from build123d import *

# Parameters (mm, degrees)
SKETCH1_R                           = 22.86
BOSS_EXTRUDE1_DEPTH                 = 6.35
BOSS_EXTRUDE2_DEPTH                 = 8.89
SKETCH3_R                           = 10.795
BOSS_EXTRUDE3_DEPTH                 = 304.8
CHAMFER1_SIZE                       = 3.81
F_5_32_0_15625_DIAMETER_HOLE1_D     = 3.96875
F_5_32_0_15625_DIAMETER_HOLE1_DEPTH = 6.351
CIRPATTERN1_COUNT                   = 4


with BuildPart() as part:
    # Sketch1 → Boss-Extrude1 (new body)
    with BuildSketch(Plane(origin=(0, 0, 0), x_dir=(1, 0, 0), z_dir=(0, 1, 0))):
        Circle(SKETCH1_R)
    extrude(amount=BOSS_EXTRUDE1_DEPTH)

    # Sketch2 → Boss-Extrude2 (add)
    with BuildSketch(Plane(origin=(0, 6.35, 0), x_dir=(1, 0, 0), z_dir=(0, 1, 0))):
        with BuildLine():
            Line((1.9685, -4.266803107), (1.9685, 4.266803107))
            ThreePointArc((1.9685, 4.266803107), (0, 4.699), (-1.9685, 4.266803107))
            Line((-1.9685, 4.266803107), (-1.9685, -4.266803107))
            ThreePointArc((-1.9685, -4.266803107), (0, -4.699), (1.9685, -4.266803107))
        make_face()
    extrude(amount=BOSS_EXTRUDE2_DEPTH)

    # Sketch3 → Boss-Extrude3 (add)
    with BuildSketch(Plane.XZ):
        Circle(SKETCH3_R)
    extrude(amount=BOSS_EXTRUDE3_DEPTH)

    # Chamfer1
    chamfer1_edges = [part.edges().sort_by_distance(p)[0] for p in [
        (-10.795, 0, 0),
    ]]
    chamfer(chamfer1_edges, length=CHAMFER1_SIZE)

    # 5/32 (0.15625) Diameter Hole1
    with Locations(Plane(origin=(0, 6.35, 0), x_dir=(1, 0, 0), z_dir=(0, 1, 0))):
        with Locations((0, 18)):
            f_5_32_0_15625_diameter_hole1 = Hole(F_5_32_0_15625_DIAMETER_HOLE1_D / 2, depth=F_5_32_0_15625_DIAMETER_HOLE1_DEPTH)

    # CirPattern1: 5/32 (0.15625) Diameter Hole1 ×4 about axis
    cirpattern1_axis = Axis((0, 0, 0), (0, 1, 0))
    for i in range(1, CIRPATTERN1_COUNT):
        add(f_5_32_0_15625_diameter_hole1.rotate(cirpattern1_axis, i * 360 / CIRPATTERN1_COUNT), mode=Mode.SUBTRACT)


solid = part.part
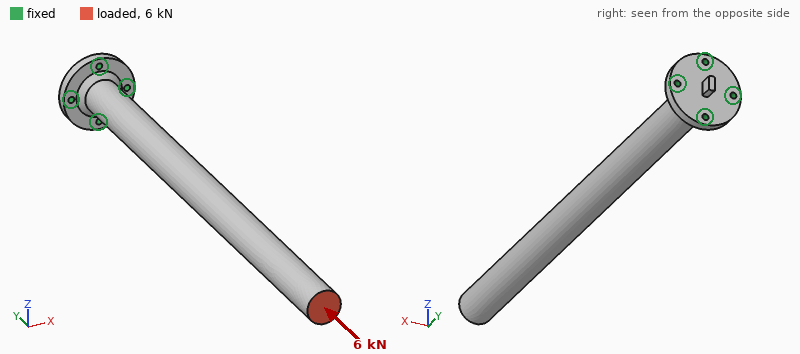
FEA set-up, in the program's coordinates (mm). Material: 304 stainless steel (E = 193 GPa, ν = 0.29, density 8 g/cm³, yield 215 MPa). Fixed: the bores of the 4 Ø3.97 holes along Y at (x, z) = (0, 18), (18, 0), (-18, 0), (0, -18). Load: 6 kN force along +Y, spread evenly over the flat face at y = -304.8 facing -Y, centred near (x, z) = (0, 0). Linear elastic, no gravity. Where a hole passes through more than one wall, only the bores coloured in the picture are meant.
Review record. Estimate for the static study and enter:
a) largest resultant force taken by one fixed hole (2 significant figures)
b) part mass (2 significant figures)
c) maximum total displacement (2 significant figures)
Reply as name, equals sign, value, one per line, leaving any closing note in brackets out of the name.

largest resultant force taken by one fixed hole = 1.6 kN
part mass = 980 g
maximum total displacement = 28 µm
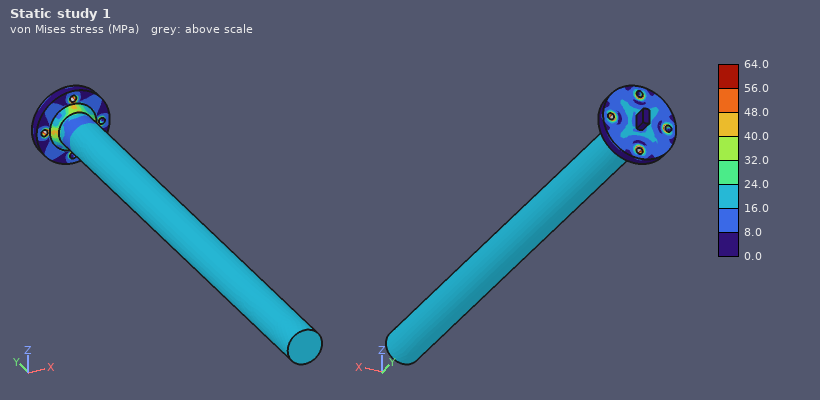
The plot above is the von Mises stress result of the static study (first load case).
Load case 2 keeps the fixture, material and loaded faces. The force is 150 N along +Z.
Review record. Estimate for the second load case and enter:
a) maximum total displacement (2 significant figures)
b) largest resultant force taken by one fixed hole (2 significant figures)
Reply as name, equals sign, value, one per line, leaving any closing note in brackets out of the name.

maximum total displacement = 0.73 mm
largest resultant force taken by one fixed hole = 1.3 kN
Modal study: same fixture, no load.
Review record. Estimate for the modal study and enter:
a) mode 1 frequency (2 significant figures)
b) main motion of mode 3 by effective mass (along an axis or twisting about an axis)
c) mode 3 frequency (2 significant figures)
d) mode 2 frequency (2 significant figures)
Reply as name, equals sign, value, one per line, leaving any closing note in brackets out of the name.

mode 1 frequency = 150 Hz
main motion of mode 3 by effective mass = along Z
mode 3 frequency = 950 Hz
mode 2 frequency = 150 Hz
